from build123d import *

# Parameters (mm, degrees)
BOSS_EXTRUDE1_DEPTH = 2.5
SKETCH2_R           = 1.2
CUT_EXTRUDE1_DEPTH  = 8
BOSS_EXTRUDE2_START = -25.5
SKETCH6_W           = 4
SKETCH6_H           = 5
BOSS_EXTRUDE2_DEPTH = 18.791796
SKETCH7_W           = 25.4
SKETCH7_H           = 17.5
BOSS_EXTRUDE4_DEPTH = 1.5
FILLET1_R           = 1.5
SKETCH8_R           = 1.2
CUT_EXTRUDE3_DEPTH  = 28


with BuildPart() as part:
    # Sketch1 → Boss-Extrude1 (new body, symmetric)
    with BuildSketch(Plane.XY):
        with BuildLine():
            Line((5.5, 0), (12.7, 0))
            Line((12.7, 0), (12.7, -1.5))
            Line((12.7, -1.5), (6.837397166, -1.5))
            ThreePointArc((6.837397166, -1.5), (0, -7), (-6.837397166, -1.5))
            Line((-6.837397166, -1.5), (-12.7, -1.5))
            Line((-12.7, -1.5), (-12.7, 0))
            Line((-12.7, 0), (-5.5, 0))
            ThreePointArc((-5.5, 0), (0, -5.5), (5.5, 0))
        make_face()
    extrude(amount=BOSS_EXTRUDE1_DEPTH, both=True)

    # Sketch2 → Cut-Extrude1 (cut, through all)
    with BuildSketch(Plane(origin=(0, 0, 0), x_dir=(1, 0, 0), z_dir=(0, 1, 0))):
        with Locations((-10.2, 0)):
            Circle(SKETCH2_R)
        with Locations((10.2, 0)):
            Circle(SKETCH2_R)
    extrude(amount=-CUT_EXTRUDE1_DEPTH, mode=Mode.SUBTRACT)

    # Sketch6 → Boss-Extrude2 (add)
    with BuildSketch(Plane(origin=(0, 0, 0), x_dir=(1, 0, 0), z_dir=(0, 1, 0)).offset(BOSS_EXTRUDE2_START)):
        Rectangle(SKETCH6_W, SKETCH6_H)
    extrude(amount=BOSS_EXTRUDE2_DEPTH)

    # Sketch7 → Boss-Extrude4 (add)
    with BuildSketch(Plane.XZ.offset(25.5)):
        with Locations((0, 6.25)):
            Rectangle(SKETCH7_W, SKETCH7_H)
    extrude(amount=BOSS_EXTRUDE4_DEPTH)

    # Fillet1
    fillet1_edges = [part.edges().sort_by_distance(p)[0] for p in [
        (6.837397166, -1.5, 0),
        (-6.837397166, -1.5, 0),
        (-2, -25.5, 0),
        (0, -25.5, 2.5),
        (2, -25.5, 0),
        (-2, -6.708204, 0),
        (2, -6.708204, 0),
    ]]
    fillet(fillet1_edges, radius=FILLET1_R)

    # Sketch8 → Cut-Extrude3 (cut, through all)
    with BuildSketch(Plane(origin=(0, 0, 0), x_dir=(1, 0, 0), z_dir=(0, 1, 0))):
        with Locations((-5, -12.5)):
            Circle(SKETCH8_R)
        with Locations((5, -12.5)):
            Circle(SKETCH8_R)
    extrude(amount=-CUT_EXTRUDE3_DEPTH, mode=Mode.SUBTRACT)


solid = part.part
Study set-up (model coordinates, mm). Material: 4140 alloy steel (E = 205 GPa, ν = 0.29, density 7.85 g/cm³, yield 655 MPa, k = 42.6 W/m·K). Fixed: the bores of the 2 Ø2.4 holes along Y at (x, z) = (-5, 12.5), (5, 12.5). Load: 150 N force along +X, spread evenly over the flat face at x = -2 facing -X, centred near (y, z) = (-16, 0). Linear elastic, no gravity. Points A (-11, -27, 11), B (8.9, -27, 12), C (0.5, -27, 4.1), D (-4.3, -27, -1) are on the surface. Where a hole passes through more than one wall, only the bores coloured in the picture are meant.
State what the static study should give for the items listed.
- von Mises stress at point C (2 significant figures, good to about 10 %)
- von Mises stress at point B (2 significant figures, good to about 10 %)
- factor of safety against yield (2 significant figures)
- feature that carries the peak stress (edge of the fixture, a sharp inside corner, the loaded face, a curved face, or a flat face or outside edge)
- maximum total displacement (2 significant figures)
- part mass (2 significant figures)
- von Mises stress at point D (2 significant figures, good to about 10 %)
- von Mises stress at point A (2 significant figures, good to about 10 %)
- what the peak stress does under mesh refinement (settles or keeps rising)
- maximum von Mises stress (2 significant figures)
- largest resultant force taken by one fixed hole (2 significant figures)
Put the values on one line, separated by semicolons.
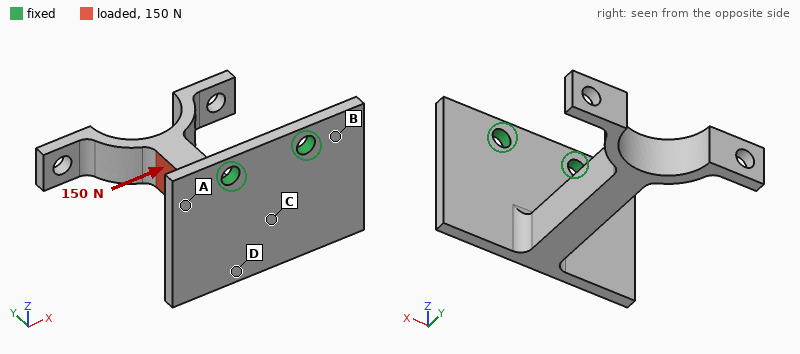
140 MPa; 79 MPa; 1.5; a curved face; 0.20 mm; 9.9 g; 120 MPa; 56 MPa; settles; 420 MPa; 210 N
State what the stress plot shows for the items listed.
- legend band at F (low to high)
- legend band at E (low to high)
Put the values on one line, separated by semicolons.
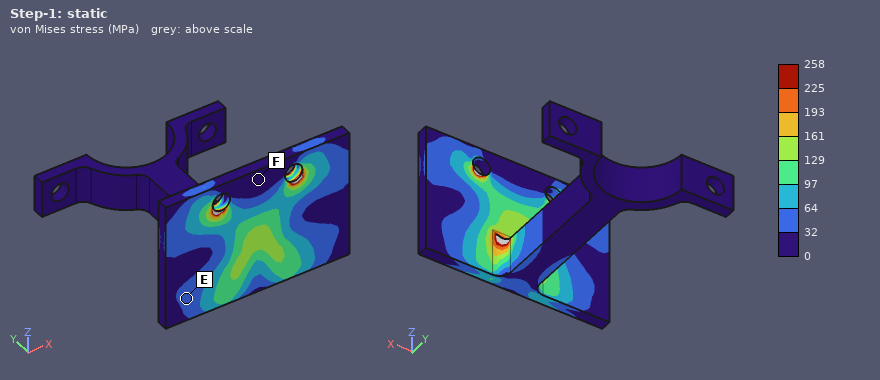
0 to 32 MPa; 32 to 64 MPa
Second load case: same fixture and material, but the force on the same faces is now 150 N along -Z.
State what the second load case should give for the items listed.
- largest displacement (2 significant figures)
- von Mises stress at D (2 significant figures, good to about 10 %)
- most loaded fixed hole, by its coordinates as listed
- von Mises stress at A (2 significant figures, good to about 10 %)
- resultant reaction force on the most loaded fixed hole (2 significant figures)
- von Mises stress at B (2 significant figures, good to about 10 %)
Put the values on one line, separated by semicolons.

0.38 mm; 90 MPa; (-5, 12.5); 94 MPa; 110 N; 99 MPa
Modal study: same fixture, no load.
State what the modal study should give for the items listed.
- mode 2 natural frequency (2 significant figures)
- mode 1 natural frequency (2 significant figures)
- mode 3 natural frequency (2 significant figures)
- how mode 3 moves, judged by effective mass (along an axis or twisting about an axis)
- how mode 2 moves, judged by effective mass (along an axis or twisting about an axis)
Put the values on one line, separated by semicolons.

1900 Hz; 1300 Hz; 5500 Hz; along Y; along X
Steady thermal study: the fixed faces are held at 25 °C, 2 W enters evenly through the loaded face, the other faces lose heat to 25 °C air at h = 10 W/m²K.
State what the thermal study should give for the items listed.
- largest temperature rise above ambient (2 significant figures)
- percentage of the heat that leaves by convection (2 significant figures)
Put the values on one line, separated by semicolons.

37 K; 14 %
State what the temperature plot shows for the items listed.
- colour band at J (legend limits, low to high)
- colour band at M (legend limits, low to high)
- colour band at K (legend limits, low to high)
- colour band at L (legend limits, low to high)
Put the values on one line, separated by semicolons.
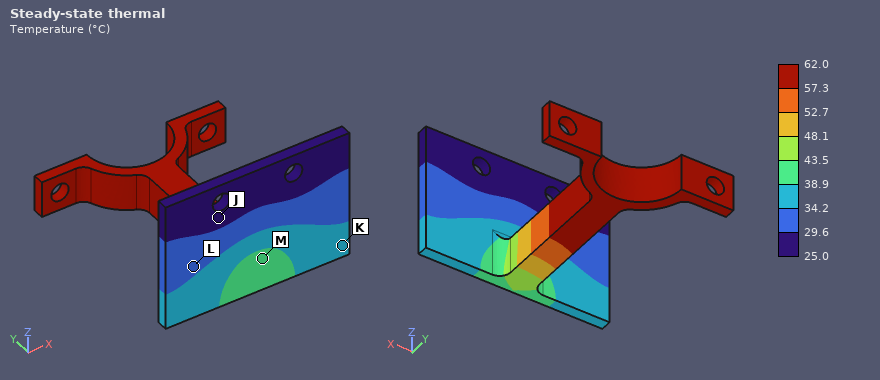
25.0 to 29.6 °C; 38.9 to 43.5 °C; 34.2 to 38.9 °C; 29.6 to 34.2 °C
